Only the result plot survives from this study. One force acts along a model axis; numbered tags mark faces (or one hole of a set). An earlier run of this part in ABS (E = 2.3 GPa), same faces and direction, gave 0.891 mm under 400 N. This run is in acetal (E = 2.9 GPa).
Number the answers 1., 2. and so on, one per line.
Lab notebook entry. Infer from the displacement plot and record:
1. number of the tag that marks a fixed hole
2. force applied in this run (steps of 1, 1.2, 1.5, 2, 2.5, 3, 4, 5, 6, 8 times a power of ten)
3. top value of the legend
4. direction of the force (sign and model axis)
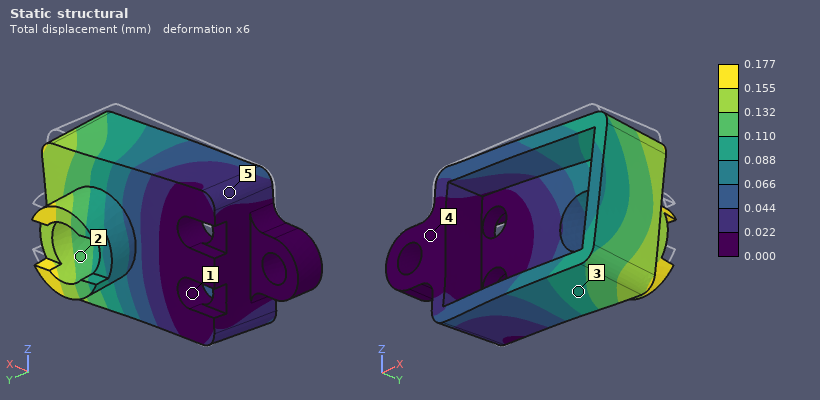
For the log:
1. 1
2. 100 N
3. 0.177 mm
4. -Z
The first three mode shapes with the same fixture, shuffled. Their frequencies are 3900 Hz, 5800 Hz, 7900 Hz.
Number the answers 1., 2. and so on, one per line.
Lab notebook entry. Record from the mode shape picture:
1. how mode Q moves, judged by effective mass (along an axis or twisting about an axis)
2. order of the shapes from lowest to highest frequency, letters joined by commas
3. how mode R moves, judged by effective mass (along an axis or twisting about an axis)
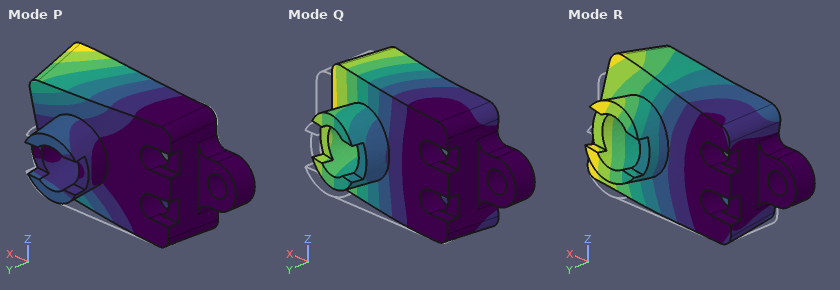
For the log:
1. along Y
2. Q, P, R
3. along Z
